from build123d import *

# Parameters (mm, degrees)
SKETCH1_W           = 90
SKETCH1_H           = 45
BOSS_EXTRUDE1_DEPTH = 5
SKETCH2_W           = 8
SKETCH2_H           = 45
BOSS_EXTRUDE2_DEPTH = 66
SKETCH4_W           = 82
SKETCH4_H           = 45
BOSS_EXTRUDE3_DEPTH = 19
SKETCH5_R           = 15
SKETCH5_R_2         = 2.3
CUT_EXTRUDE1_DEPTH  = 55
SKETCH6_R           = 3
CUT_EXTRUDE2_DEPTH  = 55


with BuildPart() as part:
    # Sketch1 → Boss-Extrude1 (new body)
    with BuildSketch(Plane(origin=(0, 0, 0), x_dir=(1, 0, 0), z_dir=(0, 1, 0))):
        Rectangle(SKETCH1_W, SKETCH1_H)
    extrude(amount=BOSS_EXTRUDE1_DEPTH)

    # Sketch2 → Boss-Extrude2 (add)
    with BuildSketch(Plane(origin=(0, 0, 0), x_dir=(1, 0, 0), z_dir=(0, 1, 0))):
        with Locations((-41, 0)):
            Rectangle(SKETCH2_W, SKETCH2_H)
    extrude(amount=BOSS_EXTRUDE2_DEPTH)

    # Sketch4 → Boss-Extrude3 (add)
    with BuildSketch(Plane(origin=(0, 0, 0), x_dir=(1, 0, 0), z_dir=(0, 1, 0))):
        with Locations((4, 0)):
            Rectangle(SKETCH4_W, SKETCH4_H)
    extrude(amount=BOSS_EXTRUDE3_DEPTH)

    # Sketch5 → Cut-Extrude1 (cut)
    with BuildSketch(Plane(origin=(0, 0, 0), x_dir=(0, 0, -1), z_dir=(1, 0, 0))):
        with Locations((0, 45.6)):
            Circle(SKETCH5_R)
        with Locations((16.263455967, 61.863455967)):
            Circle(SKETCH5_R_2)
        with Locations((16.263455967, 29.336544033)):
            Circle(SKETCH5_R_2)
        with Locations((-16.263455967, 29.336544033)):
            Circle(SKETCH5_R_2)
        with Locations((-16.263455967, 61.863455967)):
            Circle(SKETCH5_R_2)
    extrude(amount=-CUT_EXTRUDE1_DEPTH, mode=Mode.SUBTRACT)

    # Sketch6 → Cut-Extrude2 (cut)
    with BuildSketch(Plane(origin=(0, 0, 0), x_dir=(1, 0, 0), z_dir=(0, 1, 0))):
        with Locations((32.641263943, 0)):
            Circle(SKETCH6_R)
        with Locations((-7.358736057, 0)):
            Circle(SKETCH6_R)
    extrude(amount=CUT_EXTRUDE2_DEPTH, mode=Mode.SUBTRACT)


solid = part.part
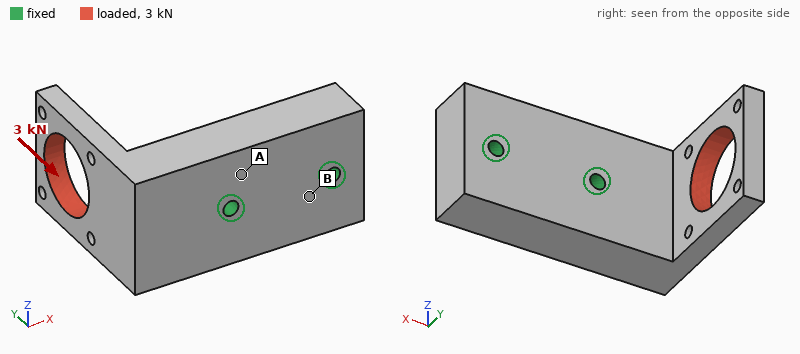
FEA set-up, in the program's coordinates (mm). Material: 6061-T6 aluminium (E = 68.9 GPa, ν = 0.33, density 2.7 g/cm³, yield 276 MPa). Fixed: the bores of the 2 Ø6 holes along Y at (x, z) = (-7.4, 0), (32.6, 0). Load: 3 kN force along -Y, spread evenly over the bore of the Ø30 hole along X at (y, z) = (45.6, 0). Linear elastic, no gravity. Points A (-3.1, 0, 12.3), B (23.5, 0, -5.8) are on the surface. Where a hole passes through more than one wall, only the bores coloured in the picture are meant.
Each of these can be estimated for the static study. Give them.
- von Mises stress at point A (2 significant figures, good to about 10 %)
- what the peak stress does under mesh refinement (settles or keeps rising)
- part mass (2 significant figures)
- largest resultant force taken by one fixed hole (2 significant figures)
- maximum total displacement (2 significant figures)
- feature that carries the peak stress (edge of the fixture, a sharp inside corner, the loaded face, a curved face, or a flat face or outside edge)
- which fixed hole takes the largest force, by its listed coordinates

18 MPa
keeps rising
230 g
3.9 kN
98 µm
edge of the fixture
(-7.4, 0)
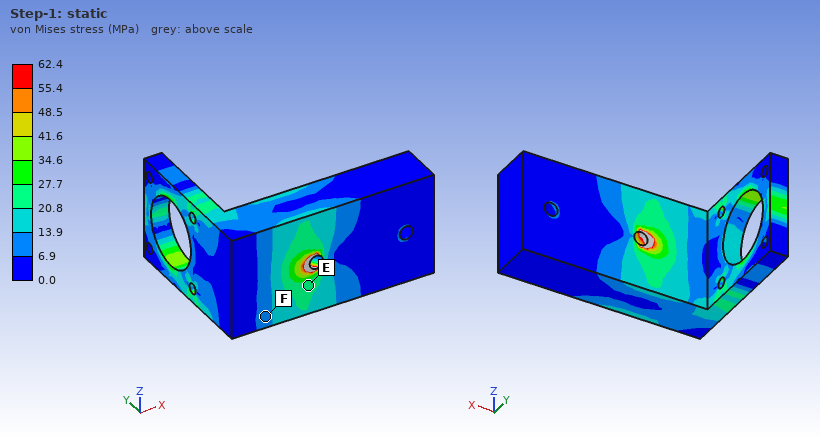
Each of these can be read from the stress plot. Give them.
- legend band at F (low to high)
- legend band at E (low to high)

6.9 to 13.9 MPa
20.8 to 27.7 MPa
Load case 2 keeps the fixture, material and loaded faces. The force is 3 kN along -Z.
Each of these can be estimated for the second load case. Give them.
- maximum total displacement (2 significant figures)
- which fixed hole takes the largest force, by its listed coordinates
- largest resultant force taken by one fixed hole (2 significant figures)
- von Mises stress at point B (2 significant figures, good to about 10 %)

0.24 mm
(-7.4, 0)
5.1 kN
14 MPa
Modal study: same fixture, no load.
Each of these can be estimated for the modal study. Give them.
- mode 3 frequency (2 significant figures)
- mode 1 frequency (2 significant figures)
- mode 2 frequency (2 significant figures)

4800 Hz
2300 Hz
4000 Hz
